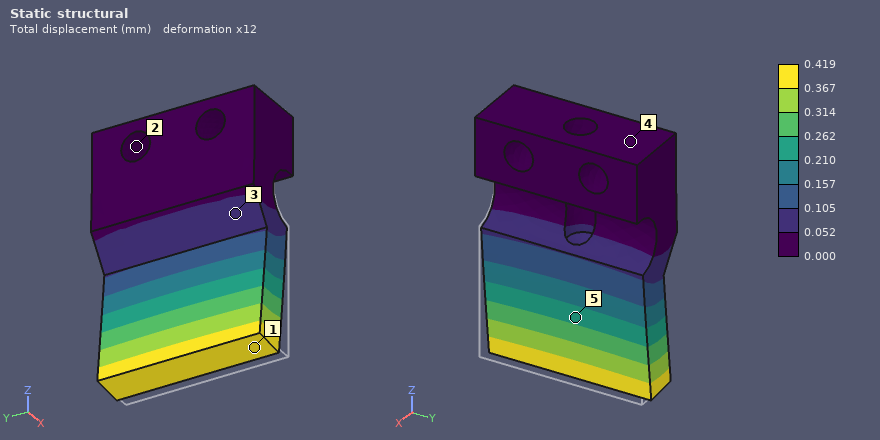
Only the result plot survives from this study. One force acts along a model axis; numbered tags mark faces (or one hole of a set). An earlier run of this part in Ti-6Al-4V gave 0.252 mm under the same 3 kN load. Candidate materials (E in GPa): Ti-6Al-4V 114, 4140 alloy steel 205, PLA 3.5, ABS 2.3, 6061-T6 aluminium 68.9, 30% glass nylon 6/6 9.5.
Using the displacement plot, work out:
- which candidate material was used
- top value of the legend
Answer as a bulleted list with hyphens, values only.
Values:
- 6061-T6 aluminium
- 0.419 mm
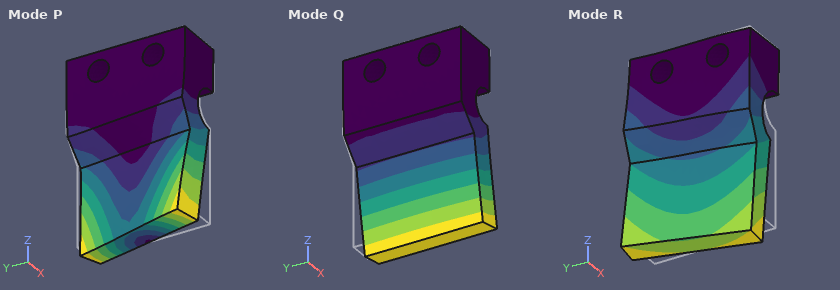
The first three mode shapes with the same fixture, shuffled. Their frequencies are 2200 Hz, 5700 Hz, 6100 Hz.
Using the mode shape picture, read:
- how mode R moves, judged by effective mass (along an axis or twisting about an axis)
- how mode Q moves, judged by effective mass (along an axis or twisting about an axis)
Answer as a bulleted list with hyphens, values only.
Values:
- along Y
- along X
